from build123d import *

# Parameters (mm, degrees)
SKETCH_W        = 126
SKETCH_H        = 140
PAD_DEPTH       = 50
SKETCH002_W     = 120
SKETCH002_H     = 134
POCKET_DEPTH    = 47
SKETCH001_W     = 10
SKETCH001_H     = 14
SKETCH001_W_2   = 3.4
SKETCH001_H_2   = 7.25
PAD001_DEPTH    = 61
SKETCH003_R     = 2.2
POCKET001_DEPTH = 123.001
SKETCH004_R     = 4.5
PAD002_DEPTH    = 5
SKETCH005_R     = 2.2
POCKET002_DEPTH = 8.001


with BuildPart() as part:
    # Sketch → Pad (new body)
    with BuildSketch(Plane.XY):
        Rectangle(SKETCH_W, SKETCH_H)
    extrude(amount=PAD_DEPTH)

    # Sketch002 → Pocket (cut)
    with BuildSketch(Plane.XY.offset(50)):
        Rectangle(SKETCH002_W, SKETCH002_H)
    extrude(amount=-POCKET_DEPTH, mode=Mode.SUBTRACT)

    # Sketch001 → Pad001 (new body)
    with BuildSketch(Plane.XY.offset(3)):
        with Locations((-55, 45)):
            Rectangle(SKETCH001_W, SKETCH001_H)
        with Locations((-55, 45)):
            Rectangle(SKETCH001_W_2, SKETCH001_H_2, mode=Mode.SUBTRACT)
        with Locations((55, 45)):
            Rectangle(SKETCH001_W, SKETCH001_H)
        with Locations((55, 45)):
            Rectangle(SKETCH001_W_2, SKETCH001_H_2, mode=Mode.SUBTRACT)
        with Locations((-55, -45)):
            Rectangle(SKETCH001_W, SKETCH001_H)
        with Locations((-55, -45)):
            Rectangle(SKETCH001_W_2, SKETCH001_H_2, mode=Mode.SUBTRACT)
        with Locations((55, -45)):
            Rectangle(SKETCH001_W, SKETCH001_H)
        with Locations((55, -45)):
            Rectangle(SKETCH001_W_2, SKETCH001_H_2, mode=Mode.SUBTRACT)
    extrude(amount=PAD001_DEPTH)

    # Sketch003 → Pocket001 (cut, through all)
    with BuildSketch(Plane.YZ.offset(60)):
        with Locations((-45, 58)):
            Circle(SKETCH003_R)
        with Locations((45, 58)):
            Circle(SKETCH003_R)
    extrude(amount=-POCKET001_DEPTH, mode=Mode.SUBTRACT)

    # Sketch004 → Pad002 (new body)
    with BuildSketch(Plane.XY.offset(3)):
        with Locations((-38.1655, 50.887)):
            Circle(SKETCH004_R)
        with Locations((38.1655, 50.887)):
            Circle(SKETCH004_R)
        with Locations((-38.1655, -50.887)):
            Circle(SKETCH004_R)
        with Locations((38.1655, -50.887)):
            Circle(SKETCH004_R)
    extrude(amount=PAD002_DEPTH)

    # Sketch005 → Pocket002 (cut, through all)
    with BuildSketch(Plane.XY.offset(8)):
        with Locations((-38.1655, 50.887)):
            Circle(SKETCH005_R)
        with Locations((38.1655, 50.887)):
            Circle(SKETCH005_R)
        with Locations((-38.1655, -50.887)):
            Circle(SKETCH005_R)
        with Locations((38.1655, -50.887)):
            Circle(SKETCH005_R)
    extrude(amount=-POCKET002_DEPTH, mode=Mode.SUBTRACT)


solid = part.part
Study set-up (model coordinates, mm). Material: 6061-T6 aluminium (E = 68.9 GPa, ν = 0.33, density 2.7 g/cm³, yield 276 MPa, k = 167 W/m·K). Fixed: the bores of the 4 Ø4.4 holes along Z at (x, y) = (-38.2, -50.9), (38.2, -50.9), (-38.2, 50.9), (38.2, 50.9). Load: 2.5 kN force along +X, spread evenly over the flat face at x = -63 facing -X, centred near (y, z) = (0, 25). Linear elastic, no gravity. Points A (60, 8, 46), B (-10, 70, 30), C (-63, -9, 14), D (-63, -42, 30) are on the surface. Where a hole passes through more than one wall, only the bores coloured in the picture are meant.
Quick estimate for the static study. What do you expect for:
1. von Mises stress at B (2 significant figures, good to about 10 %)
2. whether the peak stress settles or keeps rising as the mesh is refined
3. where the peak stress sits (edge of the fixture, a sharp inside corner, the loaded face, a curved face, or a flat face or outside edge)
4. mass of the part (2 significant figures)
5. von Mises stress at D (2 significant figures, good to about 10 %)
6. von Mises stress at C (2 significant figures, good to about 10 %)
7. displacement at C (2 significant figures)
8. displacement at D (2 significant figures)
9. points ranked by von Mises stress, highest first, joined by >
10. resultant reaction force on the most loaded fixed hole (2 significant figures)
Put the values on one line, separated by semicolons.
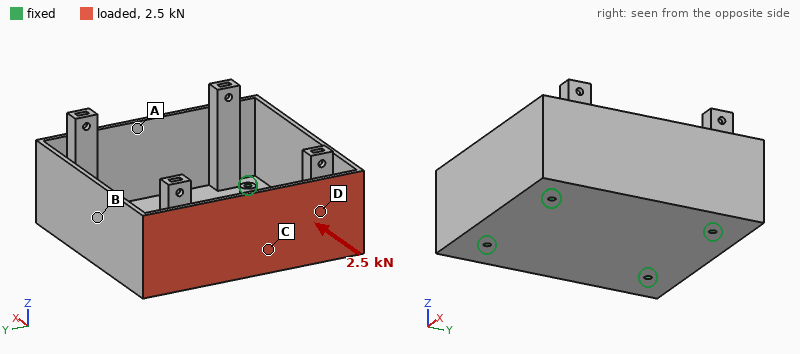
13 MPa; keeps rising; edge of the fixture; 420 g; 34 MPa; 23 MPa; 0.18 mm; 0.20 mm; D > C > B > A; 800 N
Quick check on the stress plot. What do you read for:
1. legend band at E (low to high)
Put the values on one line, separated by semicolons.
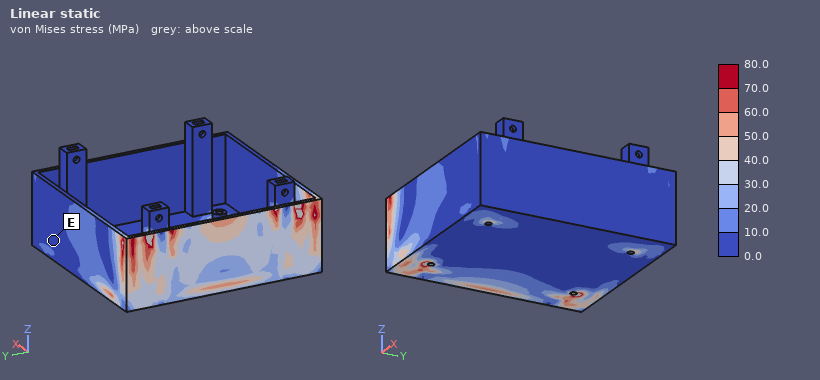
0.0 to 10.0 MPa
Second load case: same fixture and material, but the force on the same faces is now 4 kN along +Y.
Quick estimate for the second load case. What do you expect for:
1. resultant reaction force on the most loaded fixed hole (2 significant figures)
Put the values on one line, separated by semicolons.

2.3 kN
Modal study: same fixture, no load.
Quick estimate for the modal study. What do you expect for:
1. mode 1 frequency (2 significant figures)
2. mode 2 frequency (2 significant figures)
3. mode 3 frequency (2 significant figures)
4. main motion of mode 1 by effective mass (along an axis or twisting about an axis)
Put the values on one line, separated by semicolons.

1200 Hz; 1400 Hz; 1400 Hz; along X
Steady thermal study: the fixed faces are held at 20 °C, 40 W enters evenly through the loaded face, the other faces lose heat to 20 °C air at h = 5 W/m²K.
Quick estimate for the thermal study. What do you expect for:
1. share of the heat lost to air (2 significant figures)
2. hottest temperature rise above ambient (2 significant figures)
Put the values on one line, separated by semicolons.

7.8 %; 24 K
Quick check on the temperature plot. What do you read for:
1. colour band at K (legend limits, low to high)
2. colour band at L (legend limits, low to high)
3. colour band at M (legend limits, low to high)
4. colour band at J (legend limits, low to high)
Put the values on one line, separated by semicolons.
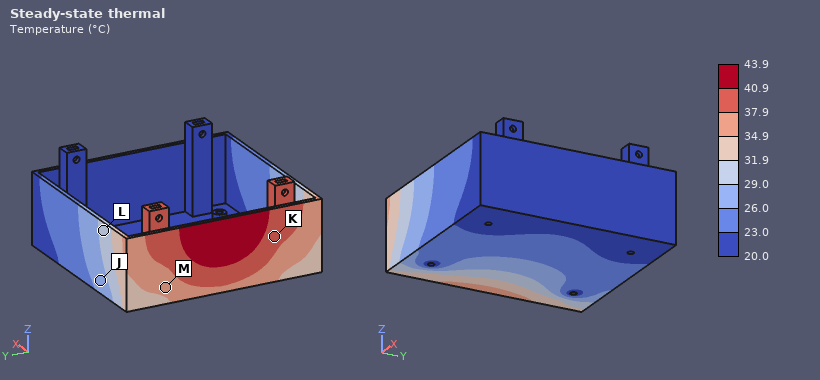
37.9 to 40.9 °C; 29.0 to 31.9 °C; 34.9 to 37.9 °C; 26.0 to 29.0 °C
